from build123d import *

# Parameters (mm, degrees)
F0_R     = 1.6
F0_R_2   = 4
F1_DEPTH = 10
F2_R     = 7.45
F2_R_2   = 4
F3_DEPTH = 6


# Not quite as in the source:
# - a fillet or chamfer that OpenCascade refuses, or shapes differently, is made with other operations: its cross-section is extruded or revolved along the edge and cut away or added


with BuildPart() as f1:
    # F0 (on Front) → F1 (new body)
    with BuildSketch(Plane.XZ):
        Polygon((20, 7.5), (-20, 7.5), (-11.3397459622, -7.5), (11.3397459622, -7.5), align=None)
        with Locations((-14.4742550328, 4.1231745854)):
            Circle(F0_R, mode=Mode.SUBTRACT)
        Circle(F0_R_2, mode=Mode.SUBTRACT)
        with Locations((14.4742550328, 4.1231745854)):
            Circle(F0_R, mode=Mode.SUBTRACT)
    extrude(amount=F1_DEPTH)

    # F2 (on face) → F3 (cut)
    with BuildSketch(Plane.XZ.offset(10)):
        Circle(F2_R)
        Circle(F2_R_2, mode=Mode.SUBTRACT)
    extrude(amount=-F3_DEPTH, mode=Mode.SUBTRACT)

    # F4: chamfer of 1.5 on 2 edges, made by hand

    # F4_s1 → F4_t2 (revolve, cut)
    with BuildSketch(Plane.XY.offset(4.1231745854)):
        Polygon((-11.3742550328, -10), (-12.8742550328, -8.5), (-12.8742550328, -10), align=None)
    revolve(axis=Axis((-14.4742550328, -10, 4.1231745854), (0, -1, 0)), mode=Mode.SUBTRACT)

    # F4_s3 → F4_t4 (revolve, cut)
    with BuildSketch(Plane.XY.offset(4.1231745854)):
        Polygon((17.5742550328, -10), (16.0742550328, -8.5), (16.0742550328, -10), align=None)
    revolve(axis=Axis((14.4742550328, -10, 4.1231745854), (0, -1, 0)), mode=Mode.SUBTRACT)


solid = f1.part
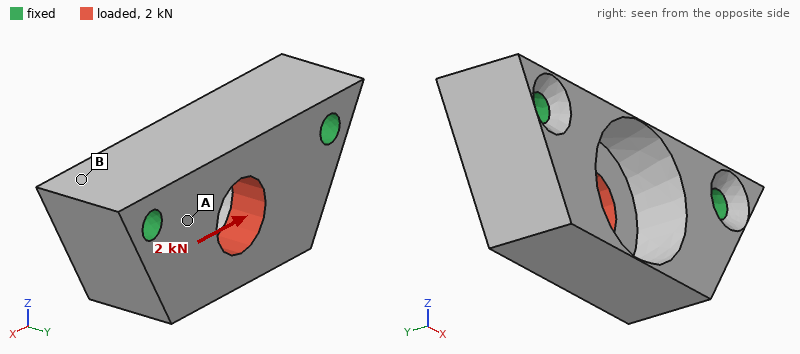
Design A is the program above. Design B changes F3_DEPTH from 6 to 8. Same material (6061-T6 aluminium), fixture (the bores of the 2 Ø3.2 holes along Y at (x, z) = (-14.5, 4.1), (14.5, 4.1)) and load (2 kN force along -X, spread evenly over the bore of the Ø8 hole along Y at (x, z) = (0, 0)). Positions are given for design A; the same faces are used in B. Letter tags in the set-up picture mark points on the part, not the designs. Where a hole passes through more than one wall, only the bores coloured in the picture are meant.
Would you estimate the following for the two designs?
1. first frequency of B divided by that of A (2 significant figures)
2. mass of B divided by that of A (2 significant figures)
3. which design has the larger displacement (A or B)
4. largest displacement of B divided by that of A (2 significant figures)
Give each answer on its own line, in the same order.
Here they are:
1.1
0.92
B
1.7
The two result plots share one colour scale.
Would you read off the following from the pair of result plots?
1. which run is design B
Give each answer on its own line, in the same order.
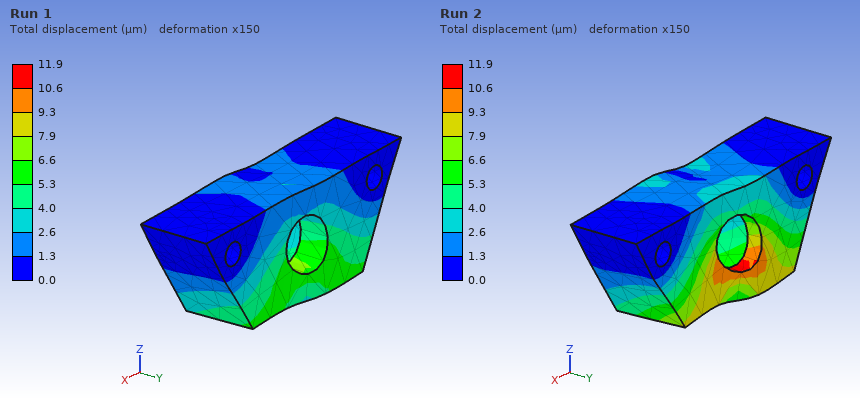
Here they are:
Run 2
